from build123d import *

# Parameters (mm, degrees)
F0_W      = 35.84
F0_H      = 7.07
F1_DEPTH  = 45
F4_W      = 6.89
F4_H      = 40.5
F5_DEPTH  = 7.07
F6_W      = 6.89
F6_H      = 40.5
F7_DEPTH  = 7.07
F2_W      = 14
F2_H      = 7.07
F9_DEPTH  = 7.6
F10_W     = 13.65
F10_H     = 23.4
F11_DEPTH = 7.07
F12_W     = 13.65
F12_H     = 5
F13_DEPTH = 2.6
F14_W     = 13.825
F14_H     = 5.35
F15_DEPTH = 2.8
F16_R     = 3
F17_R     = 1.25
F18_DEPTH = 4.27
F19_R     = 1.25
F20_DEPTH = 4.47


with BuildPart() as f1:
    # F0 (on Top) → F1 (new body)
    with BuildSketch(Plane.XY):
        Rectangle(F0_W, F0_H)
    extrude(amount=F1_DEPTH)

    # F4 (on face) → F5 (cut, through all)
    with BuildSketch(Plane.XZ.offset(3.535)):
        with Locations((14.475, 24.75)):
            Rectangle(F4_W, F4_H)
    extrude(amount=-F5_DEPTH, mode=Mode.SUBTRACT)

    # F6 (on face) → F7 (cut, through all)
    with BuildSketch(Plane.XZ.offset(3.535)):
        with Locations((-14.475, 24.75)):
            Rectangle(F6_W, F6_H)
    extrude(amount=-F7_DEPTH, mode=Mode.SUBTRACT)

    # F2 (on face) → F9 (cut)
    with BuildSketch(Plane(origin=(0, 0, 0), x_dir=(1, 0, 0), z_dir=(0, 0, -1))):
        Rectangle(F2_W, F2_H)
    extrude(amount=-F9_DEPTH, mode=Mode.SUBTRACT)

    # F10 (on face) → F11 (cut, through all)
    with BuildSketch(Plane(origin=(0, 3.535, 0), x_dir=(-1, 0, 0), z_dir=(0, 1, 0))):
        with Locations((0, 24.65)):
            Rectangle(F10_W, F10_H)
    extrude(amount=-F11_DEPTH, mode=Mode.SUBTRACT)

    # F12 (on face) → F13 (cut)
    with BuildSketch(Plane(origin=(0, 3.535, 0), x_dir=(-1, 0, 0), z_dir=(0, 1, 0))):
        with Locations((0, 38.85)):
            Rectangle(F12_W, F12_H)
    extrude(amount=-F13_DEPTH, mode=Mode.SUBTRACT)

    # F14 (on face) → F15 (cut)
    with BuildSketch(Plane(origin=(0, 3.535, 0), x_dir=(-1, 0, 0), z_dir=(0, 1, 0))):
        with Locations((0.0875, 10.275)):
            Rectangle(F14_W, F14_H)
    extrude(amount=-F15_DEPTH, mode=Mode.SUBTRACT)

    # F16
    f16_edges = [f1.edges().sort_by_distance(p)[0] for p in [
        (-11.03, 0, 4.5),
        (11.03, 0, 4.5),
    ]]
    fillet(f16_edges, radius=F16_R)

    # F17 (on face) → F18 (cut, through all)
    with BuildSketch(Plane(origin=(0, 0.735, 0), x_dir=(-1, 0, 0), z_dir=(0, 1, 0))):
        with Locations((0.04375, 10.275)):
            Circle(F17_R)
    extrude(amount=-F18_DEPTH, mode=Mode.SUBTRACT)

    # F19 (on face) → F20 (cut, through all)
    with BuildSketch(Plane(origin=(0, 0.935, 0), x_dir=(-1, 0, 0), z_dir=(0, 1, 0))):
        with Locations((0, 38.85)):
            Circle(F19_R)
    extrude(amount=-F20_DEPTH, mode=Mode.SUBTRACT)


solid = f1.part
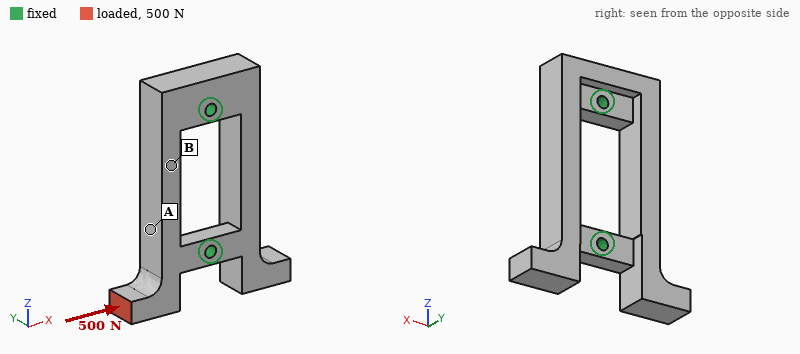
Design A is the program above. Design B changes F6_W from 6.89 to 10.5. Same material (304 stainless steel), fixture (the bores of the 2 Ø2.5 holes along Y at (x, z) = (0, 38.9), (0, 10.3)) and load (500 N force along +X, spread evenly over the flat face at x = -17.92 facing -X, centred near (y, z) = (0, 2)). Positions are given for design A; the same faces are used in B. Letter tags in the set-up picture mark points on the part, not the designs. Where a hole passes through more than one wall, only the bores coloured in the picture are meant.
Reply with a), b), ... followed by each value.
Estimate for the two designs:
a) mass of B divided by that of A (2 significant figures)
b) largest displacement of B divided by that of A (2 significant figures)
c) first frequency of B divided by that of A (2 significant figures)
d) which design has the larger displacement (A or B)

a) 0.87
b) 2.9
c) 0.84
d) B
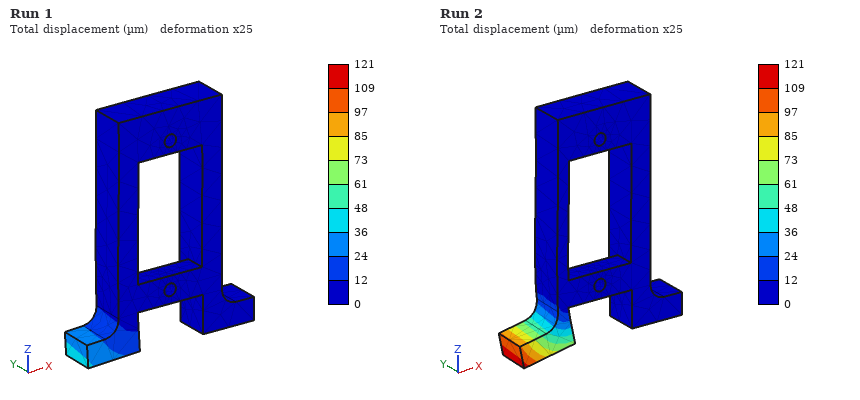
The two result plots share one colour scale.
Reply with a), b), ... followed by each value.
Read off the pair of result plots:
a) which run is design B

a) Run 2
